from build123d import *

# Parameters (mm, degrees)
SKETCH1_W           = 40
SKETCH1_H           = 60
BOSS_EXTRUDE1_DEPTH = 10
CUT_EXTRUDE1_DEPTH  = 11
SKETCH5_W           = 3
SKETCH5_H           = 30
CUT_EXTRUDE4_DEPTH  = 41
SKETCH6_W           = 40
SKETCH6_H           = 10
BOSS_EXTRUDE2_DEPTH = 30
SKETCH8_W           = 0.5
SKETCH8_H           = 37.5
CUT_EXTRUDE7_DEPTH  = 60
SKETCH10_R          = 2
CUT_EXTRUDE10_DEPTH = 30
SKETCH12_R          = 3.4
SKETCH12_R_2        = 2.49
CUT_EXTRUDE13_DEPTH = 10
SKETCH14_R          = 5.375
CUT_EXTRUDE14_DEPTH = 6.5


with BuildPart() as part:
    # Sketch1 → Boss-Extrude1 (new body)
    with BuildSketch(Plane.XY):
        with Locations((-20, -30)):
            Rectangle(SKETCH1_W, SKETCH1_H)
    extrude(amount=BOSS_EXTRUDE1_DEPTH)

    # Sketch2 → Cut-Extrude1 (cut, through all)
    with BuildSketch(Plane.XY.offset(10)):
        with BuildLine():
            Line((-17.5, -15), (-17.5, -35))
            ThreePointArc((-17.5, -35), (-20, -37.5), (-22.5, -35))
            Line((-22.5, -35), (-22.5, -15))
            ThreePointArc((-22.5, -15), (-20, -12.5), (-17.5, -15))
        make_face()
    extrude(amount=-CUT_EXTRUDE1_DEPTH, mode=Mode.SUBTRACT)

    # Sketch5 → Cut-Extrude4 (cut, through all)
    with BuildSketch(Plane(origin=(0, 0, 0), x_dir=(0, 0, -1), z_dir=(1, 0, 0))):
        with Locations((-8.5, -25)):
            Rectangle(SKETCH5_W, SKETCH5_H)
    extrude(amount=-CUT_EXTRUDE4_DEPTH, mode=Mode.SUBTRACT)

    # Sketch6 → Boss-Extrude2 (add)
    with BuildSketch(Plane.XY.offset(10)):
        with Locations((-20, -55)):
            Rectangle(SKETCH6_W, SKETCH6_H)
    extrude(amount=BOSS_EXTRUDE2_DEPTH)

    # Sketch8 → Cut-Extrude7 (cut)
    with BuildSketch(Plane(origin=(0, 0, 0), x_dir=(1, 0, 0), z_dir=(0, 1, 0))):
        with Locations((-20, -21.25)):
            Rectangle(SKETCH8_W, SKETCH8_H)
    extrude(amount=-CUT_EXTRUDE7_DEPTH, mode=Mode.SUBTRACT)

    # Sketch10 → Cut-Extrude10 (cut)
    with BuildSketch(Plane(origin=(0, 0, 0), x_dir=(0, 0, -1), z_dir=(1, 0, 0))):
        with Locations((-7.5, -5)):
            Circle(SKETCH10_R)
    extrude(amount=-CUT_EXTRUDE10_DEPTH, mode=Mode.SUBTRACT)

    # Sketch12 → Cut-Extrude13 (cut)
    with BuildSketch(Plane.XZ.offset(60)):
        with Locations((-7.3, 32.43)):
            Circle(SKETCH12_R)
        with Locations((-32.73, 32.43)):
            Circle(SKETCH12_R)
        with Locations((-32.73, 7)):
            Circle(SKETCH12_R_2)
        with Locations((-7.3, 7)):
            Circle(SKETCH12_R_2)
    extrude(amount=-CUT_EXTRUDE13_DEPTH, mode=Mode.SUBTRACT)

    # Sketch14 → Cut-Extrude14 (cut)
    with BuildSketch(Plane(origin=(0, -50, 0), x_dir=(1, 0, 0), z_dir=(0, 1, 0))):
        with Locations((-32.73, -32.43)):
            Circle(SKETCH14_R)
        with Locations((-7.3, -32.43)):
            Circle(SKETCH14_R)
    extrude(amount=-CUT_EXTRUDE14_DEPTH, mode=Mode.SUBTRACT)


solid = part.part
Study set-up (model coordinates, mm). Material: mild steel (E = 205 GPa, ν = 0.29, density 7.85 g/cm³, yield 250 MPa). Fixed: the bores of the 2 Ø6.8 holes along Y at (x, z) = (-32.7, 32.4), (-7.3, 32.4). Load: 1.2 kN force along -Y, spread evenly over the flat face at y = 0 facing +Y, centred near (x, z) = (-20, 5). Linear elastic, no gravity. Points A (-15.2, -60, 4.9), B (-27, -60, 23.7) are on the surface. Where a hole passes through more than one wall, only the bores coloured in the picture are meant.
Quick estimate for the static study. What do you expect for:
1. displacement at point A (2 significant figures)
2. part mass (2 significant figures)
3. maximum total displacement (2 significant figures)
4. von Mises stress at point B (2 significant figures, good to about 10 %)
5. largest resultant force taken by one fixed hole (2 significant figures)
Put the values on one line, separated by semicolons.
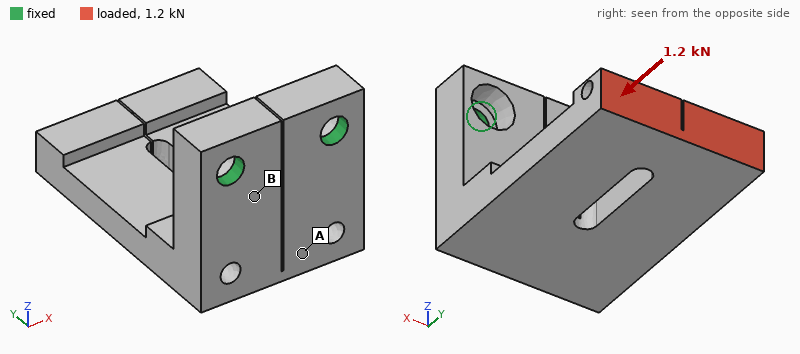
38 µm; 230 g; 98 µm; 36 MPa; 600 N
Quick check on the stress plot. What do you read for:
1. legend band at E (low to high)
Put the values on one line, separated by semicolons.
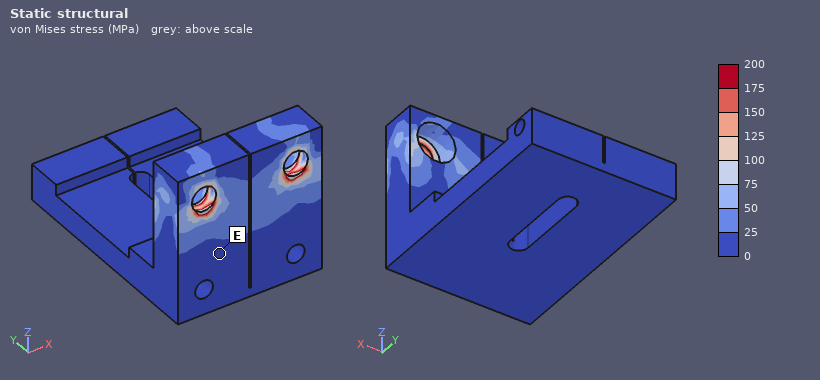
0 to 25 MPa
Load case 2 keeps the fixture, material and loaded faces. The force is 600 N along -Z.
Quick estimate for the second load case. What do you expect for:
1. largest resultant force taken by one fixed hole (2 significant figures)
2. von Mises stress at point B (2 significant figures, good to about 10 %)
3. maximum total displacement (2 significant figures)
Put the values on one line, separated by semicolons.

300 N; 53 MPa; 0.24 mm
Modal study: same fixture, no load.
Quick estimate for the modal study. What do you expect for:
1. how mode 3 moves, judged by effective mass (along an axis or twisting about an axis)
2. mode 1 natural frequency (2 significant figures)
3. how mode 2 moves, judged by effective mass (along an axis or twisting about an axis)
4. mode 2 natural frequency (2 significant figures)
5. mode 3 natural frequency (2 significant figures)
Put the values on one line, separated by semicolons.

along Y; 1200 Hz; along X; 2100 Hz; 3600 Hz
